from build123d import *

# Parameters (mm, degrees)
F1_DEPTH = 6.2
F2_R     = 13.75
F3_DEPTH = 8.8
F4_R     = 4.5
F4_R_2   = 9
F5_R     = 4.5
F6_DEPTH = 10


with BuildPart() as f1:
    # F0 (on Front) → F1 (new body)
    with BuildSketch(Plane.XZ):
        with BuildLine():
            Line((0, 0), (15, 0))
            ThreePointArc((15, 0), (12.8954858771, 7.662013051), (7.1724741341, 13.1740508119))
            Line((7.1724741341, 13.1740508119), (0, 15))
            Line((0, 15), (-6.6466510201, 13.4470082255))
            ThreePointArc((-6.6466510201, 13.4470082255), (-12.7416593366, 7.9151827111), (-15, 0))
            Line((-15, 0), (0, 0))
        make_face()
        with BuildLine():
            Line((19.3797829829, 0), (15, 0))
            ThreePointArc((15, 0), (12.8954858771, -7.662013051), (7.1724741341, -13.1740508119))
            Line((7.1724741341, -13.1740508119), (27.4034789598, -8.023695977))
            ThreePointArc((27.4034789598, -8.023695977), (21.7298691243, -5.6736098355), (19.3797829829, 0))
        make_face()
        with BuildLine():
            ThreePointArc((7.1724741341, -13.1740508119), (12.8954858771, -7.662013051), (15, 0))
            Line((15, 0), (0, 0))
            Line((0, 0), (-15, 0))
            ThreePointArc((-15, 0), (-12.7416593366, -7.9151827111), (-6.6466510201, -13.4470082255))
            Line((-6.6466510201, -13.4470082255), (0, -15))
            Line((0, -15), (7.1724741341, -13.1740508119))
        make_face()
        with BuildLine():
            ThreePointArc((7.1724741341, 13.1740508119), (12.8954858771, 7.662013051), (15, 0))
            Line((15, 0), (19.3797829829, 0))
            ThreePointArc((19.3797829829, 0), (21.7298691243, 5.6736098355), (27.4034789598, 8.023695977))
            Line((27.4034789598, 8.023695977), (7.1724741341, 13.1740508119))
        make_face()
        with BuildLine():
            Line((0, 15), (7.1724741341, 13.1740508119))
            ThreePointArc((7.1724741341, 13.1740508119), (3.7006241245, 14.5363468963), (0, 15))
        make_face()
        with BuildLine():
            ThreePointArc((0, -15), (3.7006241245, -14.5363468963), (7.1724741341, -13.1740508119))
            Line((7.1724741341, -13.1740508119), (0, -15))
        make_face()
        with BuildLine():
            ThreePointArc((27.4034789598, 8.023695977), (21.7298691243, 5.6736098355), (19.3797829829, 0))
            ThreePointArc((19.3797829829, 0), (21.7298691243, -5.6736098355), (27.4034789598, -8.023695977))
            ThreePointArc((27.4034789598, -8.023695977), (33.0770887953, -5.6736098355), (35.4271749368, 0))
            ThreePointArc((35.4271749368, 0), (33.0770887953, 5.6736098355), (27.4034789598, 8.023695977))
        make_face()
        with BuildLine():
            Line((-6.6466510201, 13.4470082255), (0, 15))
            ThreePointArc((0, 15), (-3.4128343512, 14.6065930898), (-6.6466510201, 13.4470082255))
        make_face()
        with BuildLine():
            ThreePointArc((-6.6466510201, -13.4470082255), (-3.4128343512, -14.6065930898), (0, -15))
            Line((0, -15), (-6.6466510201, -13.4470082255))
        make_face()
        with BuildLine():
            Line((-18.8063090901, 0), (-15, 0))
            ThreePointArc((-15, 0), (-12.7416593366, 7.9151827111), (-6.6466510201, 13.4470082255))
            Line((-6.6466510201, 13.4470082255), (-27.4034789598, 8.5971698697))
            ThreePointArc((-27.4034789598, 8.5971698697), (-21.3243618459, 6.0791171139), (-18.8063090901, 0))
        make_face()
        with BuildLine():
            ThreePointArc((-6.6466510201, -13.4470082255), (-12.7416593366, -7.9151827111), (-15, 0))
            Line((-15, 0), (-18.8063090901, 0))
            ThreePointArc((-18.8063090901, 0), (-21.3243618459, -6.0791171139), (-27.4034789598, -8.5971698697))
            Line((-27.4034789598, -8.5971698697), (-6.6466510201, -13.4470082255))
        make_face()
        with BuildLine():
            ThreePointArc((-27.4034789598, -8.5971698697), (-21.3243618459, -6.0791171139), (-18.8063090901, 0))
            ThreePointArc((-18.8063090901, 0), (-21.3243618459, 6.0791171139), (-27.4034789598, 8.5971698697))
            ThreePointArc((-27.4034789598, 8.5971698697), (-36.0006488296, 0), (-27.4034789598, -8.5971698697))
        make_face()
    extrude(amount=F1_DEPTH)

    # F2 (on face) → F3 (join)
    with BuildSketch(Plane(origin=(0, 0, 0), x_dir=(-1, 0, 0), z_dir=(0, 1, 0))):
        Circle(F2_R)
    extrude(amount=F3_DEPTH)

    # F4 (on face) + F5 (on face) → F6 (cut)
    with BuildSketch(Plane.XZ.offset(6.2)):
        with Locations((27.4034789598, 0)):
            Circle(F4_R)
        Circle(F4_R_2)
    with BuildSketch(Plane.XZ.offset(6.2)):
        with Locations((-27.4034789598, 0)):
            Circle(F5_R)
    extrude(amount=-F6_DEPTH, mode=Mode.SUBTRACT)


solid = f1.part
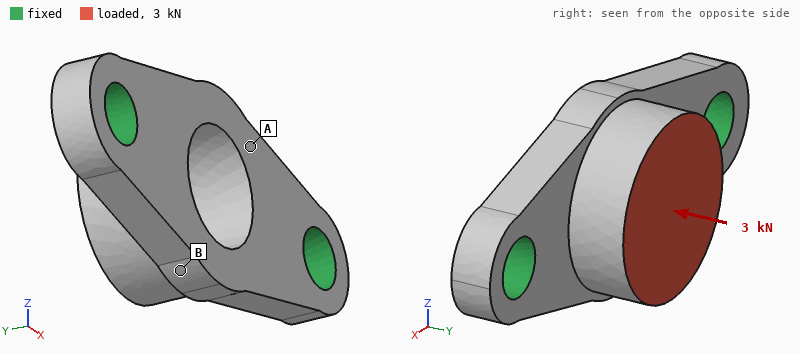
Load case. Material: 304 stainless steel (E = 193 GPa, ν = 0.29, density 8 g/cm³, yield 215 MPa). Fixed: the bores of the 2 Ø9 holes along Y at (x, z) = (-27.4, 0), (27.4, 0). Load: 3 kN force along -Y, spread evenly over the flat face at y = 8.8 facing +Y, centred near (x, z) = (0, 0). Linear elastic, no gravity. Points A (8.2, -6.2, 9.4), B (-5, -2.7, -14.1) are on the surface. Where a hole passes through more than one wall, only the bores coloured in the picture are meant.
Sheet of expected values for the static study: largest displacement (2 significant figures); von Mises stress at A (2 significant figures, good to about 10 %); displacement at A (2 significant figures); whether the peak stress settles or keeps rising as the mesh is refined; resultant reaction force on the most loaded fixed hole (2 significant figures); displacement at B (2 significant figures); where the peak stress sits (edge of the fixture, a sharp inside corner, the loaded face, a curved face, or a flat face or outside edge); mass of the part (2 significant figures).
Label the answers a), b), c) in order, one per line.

a) 11 µm
b) 31 MPa
c) 9.3 µm
d) keeps rising
e) 1.9 kN
f) 10 µm
g) edge of the fixture
h) 90 g
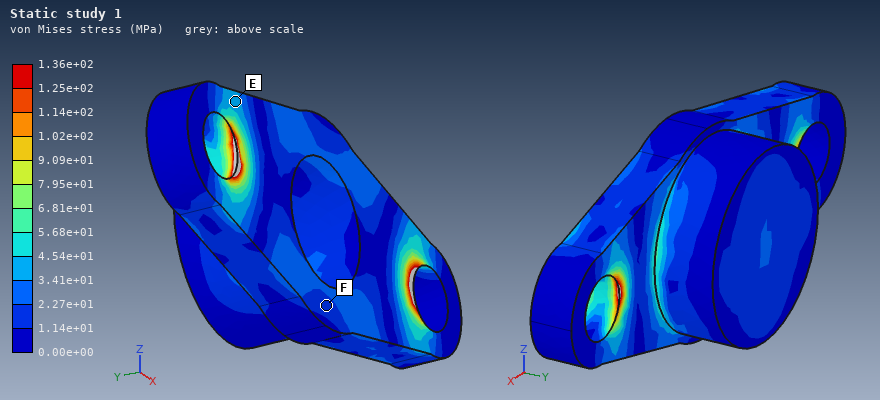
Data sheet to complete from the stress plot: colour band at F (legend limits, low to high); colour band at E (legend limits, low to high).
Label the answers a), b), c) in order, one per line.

a) 1.14e+01 to 2.27e+01 MPa
b) 3.41e+01 to 4.54e+01 MPa
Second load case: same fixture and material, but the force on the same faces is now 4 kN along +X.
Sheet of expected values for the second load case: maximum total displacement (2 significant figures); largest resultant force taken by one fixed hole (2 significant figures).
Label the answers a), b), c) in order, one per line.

a) 8.9 µm
b) 2.4 kN
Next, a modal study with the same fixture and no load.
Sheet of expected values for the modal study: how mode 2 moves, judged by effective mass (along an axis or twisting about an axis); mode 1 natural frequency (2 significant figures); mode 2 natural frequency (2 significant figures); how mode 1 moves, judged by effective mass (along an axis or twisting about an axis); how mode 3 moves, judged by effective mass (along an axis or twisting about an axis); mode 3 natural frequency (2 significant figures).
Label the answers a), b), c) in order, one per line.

a) along Y
b) 8200 Hz
c) 11 kHz
d) along Z
e) along Z
f) 20 kHz
